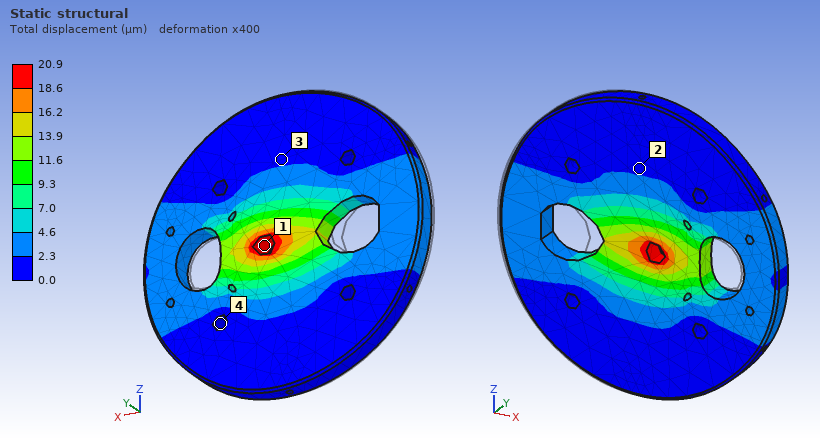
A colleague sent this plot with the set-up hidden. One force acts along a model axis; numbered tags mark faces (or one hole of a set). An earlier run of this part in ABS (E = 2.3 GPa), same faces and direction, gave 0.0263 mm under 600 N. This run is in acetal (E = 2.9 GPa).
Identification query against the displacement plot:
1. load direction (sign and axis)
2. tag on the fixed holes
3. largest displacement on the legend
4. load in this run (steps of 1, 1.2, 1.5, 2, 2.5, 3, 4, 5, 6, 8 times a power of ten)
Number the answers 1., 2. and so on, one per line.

1. +X
2. 4
3. 20.9 µm
4. 600 N
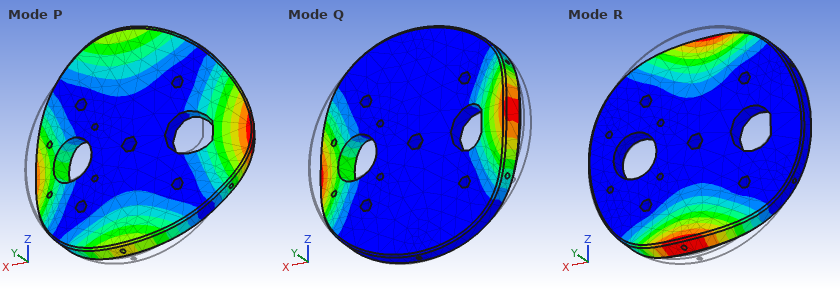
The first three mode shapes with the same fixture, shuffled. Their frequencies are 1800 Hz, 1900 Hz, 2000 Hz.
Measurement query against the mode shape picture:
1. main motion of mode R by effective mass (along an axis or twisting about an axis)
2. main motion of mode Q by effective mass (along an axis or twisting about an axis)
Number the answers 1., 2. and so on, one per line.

1. twisting about X
2. twisting about Z
